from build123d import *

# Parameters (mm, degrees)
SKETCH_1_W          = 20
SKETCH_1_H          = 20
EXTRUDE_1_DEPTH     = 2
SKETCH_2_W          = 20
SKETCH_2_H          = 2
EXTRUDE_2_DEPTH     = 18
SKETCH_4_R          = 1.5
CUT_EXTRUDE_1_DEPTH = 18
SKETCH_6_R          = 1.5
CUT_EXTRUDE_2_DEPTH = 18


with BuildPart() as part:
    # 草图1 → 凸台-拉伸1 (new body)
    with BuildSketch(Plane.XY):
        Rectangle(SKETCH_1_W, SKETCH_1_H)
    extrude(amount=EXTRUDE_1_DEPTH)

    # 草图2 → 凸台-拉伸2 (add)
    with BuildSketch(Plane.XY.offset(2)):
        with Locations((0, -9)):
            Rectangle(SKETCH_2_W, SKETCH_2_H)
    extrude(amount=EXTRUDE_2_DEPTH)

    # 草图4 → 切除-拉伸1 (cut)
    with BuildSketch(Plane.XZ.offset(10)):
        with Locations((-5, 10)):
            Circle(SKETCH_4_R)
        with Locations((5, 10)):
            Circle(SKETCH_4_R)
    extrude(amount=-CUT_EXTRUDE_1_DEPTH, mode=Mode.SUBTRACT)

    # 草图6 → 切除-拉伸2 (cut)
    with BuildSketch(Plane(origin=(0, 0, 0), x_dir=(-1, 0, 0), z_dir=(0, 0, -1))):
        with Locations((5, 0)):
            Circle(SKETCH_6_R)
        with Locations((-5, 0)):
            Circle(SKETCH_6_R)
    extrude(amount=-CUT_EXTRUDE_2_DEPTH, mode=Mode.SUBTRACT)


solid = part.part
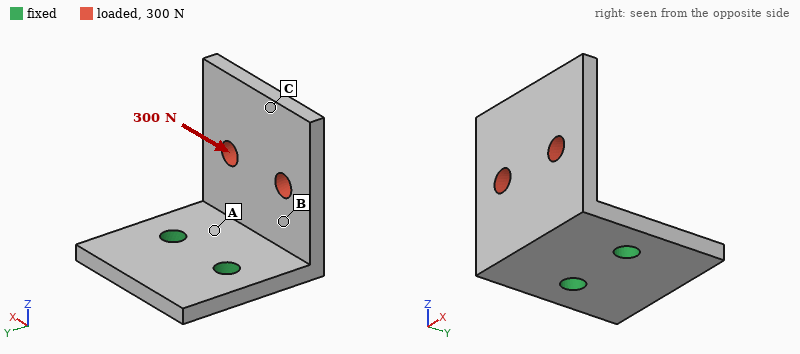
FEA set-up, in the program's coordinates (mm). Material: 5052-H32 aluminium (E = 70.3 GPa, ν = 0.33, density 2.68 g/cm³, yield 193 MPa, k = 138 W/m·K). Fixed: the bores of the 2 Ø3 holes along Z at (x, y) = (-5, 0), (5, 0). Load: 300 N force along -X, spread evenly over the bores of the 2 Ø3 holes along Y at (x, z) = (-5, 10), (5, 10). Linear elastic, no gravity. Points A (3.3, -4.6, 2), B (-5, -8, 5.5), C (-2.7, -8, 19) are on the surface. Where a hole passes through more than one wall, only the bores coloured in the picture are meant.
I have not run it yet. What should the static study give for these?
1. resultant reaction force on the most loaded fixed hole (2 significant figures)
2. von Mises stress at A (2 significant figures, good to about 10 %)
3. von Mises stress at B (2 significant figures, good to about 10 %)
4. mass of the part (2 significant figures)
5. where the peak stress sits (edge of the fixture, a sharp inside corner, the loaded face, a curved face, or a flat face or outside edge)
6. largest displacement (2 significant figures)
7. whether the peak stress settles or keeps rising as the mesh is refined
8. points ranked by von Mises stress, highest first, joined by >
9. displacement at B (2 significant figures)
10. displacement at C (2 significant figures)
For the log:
330 N
95 MPa
50 MPa
3.9 g
edge of the fixture
0.14 mm
keeps rising
A > B > C
0.045 mm
0.12 mm
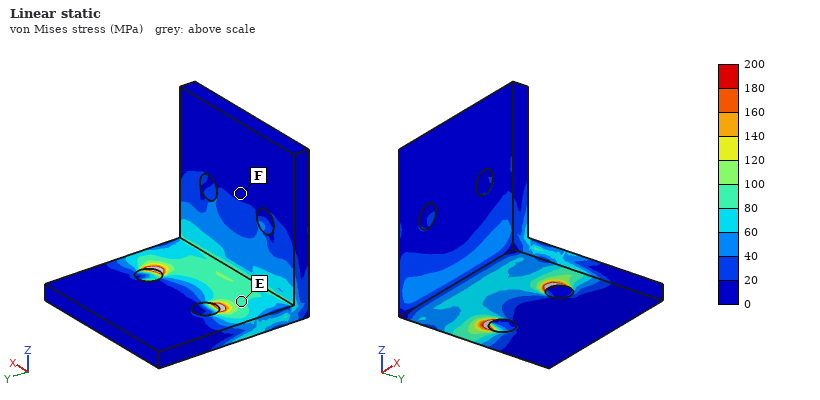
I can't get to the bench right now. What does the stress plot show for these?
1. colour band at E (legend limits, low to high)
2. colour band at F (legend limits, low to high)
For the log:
80 to 100 MPa
0 to 20 MPa
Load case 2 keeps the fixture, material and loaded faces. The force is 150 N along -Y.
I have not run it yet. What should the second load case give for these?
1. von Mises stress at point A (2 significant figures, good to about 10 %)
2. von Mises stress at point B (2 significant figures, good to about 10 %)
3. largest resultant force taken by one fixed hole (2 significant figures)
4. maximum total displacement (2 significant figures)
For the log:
97 MPa
47 MPa
78 N
0.30 mm
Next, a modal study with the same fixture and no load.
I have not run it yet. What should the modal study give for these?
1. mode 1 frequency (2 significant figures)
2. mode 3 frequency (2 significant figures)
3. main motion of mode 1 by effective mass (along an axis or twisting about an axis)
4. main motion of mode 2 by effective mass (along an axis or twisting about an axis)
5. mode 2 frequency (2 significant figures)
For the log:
2800 Hz
9800 Hz
along Y
along X
5700 Hz
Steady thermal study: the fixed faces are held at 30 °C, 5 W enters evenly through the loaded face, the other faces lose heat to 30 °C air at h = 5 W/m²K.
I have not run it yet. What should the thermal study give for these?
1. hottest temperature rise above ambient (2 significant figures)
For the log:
17 K
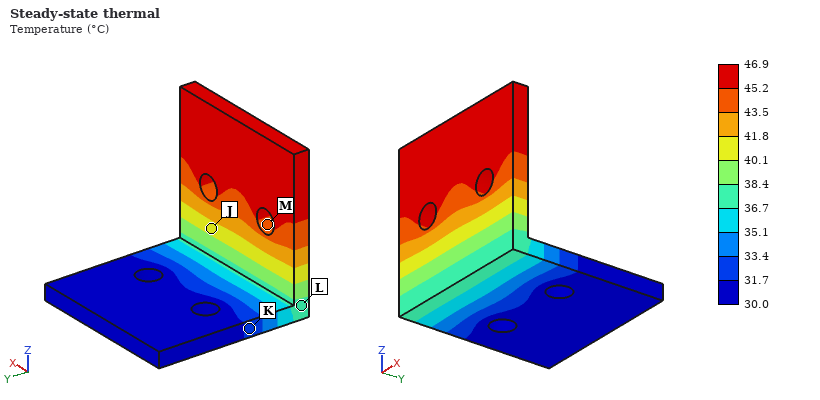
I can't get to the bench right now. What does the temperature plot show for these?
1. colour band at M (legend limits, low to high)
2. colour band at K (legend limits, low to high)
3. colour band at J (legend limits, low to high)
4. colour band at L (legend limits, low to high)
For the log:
43.5 to 45.2 °C
31.7 to 33.4 °C
40.1 to 41.8 °C
36.7 to 38.4 °C
